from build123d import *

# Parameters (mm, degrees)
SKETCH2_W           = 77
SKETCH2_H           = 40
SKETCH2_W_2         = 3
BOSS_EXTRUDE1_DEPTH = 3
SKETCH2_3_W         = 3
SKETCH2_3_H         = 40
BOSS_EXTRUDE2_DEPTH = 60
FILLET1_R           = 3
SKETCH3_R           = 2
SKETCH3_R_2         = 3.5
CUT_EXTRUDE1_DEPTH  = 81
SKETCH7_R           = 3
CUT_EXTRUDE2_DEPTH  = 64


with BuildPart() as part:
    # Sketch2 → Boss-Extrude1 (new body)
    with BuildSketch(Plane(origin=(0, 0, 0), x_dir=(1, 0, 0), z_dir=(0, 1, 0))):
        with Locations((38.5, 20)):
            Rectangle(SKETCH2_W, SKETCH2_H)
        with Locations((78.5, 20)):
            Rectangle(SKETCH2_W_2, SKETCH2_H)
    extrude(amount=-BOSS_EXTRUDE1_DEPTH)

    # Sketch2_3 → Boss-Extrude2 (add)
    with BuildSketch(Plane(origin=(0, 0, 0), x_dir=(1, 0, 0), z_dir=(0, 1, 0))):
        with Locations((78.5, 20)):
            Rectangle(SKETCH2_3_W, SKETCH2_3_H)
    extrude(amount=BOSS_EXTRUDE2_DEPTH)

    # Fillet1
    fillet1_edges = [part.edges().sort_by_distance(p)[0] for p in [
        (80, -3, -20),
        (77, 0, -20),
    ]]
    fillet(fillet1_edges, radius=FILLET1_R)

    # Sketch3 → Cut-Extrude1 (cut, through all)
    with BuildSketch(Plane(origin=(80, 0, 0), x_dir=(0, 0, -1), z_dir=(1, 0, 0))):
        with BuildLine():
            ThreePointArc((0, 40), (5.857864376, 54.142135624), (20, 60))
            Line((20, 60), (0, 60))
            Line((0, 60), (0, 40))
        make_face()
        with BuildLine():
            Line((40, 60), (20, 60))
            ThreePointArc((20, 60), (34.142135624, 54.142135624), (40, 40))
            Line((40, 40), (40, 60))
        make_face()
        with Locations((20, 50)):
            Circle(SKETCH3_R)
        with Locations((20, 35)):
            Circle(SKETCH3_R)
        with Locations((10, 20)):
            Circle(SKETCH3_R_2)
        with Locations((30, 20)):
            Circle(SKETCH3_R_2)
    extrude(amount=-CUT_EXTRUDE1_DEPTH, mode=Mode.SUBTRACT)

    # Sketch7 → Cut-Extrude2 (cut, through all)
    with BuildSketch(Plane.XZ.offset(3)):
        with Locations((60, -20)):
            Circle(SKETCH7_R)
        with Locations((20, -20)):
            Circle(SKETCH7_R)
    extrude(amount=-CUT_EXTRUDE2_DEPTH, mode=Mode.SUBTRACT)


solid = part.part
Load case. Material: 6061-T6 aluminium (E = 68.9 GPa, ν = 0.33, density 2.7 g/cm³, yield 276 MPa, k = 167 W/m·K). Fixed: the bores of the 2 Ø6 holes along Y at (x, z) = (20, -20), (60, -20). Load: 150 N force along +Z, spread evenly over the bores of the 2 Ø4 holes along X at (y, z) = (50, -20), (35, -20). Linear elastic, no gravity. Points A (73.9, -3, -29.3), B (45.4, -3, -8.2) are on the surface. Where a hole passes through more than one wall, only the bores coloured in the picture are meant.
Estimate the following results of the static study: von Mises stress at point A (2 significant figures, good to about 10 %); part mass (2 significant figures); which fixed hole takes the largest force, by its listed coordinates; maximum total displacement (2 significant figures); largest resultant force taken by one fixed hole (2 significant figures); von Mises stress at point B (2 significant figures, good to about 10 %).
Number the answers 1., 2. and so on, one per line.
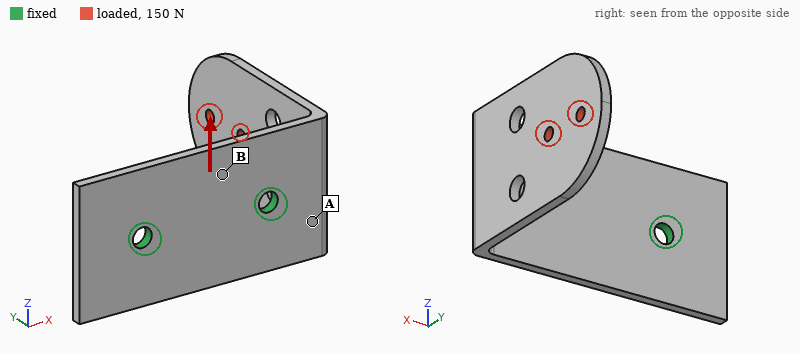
1. 44 MPa
2. 43 g
3. (60, -20)
4. 0.60 mm
5. 200 N
6. 20 MPa
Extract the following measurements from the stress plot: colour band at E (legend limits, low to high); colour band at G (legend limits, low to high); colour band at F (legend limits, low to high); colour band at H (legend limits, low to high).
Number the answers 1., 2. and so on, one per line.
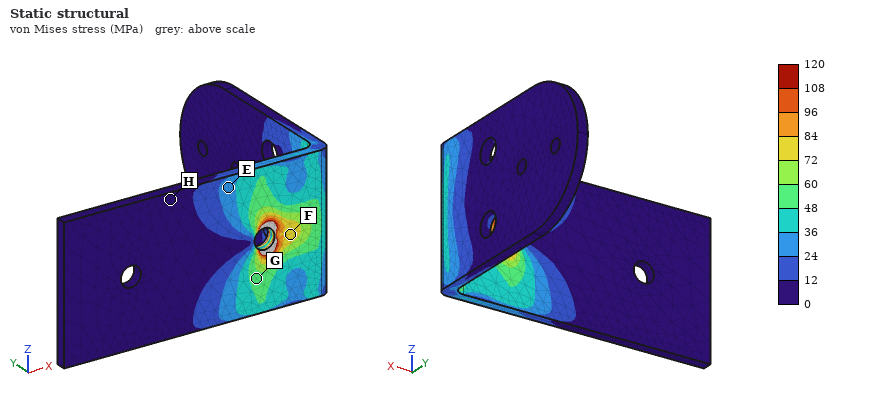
1. 24 to 36 MPa
2. 48 to 60 MPa
3. 72 to 84 MPa
4. 0 to 12 MPa
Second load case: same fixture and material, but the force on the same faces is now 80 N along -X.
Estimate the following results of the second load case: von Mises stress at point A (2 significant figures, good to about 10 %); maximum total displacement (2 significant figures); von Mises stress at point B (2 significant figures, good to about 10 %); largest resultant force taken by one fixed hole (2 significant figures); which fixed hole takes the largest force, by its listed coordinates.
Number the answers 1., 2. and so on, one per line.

1. 52 MPa
2. 1.1 mm
3. 5.9 MPa
4. 74 N
5. (60, -20)
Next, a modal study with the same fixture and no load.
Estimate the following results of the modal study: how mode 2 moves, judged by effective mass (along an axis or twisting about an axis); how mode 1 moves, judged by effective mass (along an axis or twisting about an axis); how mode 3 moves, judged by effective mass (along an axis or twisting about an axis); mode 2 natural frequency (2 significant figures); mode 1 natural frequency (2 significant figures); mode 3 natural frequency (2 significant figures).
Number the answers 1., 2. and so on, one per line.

1. along Z
2. along X
3. along Y
4. 880 Hz
5. 520 Hz
6. 2300 Hz
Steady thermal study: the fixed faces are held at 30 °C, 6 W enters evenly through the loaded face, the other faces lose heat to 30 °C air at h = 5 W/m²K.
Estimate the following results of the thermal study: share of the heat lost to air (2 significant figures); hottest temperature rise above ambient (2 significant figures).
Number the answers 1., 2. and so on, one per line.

1. 6.4 %
2. 21 K
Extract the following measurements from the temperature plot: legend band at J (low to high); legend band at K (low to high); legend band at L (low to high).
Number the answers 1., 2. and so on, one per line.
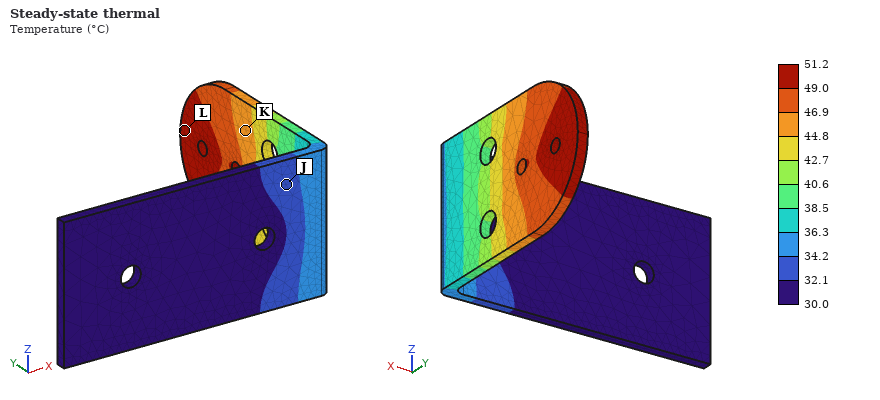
1. 32.1 to 34.2 °C
2. 44.8 to 46.9 °C
3. 49.0 to 51.2 °C
